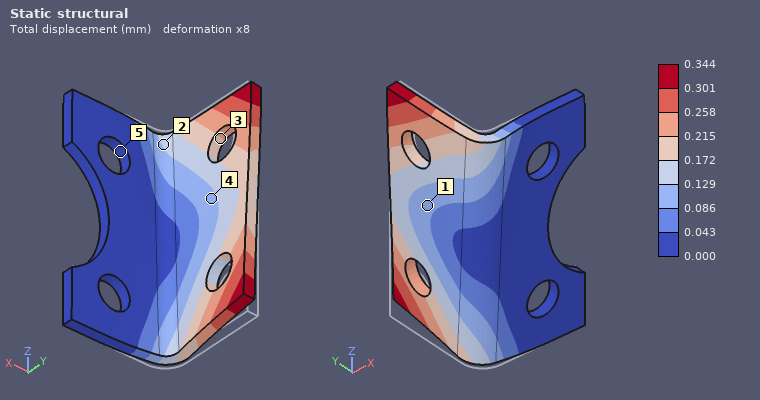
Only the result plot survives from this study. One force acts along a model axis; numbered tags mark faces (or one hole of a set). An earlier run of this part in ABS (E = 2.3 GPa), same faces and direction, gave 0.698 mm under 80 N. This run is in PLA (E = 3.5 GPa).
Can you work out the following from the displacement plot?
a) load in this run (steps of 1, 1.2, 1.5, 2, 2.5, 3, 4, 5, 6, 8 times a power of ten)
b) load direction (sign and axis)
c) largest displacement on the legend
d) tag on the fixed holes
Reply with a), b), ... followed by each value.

a) 60 N
b) +Z
c) 0.344 mm
d) 5
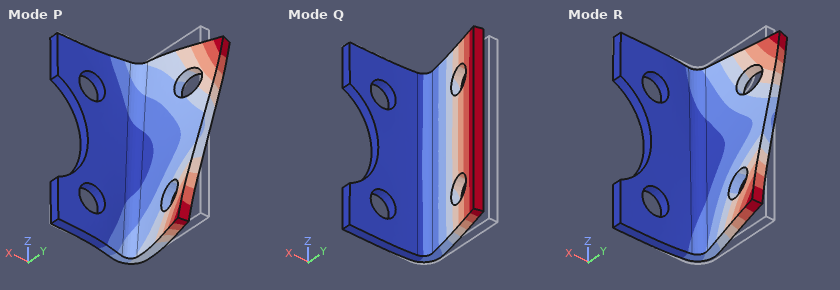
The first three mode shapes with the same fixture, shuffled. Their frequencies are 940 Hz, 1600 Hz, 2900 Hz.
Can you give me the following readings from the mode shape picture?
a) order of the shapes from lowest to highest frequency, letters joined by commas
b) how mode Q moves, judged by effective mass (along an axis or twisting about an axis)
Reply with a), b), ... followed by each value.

a) Q, R, P
b) along X
